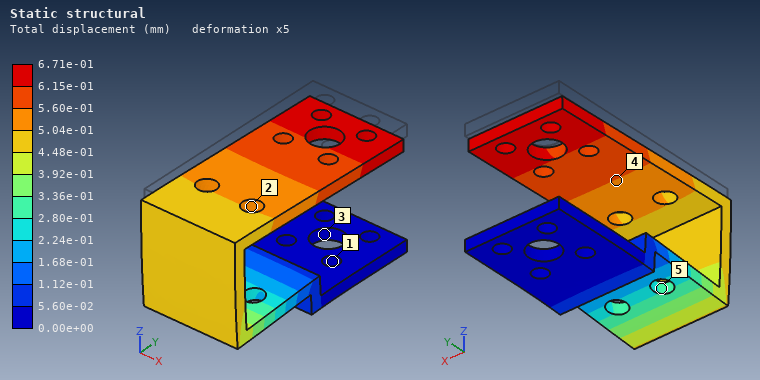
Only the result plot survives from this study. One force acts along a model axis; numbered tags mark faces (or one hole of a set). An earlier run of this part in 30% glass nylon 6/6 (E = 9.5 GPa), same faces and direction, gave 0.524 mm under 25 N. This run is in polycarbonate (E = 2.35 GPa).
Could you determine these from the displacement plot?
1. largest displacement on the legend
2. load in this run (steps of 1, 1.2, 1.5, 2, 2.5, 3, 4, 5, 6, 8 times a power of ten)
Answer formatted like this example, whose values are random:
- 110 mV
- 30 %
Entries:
- 6.71e-01 mm
- 8 N
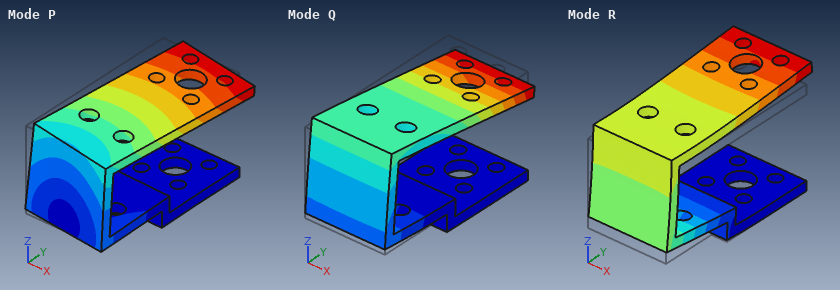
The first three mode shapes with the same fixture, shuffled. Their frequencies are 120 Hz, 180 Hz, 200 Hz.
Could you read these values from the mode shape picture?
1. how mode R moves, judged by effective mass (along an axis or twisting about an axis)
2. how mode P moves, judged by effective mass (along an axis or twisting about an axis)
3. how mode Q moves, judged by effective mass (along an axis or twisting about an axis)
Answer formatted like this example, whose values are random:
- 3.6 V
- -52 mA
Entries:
- along Z
- along X
- along Y
